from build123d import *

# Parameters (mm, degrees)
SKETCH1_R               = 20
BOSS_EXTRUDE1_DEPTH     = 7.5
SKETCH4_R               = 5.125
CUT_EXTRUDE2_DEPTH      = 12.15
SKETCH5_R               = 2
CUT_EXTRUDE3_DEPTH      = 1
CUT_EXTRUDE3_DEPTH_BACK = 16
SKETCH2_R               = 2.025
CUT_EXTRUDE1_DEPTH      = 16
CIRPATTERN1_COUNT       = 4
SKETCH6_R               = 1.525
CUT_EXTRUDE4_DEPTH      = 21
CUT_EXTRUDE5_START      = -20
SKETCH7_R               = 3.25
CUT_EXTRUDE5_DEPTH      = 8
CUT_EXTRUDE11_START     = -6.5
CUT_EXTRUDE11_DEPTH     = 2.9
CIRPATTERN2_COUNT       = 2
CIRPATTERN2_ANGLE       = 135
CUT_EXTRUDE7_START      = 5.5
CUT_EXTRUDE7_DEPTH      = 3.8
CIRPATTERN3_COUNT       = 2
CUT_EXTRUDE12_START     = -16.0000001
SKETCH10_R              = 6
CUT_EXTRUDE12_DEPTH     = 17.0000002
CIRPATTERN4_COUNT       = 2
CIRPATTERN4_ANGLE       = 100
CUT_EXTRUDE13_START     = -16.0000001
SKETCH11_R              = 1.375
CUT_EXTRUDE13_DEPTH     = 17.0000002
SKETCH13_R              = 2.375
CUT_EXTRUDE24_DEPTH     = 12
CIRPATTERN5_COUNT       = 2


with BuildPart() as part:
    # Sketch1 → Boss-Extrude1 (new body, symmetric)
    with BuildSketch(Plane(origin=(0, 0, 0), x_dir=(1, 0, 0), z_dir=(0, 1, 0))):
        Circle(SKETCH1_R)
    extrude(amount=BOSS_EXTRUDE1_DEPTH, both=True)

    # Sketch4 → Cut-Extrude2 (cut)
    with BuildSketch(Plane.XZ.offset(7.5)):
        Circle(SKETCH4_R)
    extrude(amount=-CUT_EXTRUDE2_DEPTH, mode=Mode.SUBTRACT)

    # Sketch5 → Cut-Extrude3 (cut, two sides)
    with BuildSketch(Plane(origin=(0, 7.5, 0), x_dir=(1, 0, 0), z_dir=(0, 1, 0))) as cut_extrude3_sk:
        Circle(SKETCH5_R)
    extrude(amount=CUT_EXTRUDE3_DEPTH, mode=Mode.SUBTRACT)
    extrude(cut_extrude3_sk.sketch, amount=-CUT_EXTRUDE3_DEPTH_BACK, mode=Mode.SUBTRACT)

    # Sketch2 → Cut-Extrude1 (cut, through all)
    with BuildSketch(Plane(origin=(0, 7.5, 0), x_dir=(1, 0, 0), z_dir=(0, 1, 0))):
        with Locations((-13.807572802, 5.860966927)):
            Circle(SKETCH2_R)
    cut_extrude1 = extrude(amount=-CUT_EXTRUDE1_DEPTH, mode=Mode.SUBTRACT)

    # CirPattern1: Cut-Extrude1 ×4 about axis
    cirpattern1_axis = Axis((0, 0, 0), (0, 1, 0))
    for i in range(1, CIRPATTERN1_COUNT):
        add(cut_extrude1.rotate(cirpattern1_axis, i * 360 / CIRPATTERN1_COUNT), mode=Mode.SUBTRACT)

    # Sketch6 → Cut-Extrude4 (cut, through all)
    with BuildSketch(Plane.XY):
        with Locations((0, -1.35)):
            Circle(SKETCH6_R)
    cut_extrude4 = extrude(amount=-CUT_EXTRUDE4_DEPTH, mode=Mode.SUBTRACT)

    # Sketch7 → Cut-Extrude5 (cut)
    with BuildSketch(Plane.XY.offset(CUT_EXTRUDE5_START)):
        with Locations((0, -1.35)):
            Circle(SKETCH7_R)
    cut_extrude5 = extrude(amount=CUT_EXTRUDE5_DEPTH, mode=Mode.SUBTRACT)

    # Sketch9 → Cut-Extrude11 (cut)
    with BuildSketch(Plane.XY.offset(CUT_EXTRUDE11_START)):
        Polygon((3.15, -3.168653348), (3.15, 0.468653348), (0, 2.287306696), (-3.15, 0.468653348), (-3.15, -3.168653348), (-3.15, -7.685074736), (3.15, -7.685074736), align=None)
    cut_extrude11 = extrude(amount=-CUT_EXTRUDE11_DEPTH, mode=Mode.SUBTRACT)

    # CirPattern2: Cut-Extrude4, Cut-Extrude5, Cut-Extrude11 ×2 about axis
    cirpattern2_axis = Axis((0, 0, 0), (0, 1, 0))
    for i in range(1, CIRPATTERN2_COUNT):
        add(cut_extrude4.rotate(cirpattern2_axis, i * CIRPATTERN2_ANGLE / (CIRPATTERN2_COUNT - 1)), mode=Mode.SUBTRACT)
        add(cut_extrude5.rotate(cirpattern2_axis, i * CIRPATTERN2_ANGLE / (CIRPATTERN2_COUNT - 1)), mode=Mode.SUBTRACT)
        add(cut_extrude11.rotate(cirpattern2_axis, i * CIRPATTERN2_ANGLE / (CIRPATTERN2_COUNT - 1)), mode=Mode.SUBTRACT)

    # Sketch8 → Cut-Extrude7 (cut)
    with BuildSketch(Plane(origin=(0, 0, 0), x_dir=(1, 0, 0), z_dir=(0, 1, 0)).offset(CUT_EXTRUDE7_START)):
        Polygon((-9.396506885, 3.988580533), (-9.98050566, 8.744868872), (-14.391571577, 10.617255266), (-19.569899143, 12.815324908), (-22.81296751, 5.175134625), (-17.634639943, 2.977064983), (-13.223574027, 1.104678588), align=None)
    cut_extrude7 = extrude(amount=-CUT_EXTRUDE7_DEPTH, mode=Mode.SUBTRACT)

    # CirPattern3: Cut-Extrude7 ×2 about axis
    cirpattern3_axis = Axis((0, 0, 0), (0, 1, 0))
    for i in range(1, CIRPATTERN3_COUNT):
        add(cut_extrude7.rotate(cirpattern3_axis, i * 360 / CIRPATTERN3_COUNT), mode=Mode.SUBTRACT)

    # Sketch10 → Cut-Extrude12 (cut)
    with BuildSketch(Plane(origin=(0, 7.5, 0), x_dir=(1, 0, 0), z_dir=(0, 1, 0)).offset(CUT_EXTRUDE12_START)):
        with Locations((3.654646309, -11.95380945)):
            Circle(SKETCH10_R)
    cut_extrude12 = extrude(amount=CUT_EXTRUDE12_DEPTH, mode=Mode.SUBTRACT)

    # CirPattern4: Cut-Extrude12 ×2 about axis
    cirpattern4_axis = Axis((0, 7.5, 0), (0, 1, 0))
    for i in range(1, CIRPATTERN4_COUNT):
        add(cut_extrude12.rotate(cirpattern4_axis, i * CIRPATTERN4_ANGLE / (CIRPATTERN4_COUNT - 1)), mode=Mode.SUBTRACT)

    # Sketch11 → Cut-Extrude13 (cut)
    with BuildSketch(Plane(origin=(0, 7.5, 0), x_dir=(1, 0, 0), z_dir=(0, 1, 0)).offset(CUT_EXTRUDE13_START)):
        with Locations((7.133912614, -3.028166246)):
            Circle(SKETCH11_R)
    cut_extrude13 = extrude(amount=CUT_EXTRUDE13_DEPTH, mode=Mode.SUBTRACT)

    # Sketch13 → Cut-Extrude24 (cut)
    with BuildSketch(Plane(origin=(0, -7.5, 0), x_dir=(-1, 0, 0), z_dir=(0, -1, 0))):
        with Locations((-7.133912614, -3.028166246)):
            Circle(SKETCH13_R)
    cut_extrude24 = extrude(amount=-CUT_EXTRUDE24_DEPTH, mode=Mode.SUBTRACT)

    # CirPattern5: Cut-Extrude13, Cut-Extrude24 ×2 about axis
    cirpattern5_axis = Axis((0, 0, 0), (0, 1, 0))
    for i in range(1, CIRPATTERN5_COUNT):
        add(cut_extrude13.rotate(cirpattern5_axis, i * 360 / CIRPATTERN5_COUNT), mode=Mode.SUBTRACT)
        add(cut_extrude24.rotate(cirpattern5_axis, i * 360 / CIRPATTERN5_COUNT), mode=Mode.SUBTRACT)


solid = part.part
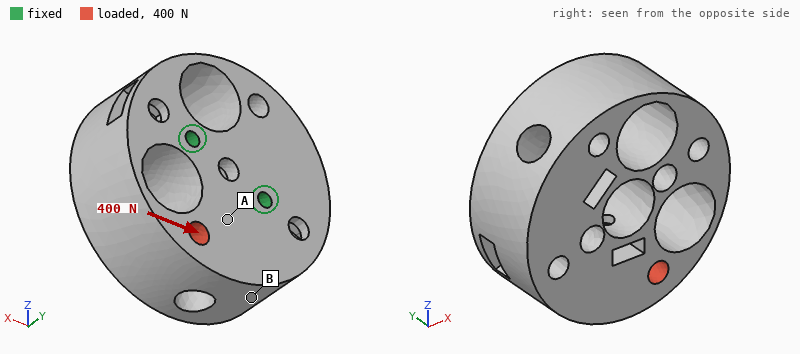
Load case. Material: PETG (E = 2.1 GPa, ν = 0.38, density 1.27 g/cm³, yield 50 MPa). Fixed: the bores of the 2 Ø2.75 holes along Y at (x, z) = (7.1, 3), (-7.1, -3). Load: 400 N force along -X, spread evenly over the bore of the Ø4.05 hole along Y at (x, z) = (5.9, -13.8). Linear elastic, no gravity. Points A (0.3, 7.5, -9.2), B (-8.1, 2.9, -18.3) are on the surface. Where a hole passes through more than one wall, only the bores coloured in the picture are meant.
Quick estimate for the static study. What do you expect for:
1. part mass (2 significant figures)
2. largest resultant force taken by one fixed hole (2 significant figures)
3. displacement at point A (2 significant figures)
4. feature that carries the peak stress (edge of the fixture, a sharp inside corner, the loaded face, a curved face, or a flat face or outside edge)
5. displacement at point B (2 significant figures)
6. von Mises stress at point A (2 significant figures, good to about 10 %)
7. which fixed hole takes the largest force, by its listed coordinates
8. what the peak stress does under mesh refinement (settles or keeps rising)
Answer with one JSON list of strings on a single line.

["15 g", "470 N", "0.13 mm", "edge of the fixture", "0.22 mm", "6.5 MPa", "(-7.1, -3)", "keeps rising"]
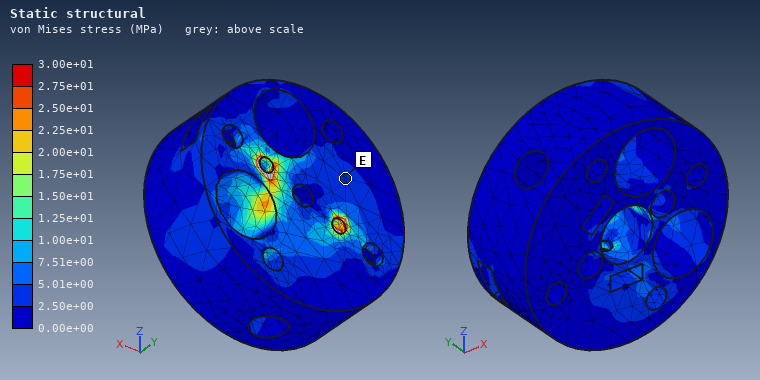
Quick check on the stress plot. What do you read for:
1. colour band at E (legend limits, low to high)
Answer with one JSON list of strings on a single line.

["2.50e+00 to 5.01e+00 MPa"]
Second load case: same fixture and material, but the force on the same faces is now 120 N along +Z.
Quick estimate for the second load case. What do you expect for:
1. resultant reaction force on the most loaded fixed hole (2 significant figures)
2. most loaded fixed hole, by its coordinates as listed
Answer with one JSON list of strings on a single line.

["100 N", "(7.1, 3)"]
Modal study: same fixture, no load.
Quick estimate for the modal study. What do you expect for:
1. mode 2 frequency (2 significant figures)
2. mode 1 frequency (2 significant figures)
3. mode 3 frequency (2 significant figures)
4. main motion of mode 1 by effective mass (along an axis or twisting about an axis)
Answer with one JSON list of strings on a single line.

["2500 Hz", "920 Hz", "2500 Hz", "along Z"]
